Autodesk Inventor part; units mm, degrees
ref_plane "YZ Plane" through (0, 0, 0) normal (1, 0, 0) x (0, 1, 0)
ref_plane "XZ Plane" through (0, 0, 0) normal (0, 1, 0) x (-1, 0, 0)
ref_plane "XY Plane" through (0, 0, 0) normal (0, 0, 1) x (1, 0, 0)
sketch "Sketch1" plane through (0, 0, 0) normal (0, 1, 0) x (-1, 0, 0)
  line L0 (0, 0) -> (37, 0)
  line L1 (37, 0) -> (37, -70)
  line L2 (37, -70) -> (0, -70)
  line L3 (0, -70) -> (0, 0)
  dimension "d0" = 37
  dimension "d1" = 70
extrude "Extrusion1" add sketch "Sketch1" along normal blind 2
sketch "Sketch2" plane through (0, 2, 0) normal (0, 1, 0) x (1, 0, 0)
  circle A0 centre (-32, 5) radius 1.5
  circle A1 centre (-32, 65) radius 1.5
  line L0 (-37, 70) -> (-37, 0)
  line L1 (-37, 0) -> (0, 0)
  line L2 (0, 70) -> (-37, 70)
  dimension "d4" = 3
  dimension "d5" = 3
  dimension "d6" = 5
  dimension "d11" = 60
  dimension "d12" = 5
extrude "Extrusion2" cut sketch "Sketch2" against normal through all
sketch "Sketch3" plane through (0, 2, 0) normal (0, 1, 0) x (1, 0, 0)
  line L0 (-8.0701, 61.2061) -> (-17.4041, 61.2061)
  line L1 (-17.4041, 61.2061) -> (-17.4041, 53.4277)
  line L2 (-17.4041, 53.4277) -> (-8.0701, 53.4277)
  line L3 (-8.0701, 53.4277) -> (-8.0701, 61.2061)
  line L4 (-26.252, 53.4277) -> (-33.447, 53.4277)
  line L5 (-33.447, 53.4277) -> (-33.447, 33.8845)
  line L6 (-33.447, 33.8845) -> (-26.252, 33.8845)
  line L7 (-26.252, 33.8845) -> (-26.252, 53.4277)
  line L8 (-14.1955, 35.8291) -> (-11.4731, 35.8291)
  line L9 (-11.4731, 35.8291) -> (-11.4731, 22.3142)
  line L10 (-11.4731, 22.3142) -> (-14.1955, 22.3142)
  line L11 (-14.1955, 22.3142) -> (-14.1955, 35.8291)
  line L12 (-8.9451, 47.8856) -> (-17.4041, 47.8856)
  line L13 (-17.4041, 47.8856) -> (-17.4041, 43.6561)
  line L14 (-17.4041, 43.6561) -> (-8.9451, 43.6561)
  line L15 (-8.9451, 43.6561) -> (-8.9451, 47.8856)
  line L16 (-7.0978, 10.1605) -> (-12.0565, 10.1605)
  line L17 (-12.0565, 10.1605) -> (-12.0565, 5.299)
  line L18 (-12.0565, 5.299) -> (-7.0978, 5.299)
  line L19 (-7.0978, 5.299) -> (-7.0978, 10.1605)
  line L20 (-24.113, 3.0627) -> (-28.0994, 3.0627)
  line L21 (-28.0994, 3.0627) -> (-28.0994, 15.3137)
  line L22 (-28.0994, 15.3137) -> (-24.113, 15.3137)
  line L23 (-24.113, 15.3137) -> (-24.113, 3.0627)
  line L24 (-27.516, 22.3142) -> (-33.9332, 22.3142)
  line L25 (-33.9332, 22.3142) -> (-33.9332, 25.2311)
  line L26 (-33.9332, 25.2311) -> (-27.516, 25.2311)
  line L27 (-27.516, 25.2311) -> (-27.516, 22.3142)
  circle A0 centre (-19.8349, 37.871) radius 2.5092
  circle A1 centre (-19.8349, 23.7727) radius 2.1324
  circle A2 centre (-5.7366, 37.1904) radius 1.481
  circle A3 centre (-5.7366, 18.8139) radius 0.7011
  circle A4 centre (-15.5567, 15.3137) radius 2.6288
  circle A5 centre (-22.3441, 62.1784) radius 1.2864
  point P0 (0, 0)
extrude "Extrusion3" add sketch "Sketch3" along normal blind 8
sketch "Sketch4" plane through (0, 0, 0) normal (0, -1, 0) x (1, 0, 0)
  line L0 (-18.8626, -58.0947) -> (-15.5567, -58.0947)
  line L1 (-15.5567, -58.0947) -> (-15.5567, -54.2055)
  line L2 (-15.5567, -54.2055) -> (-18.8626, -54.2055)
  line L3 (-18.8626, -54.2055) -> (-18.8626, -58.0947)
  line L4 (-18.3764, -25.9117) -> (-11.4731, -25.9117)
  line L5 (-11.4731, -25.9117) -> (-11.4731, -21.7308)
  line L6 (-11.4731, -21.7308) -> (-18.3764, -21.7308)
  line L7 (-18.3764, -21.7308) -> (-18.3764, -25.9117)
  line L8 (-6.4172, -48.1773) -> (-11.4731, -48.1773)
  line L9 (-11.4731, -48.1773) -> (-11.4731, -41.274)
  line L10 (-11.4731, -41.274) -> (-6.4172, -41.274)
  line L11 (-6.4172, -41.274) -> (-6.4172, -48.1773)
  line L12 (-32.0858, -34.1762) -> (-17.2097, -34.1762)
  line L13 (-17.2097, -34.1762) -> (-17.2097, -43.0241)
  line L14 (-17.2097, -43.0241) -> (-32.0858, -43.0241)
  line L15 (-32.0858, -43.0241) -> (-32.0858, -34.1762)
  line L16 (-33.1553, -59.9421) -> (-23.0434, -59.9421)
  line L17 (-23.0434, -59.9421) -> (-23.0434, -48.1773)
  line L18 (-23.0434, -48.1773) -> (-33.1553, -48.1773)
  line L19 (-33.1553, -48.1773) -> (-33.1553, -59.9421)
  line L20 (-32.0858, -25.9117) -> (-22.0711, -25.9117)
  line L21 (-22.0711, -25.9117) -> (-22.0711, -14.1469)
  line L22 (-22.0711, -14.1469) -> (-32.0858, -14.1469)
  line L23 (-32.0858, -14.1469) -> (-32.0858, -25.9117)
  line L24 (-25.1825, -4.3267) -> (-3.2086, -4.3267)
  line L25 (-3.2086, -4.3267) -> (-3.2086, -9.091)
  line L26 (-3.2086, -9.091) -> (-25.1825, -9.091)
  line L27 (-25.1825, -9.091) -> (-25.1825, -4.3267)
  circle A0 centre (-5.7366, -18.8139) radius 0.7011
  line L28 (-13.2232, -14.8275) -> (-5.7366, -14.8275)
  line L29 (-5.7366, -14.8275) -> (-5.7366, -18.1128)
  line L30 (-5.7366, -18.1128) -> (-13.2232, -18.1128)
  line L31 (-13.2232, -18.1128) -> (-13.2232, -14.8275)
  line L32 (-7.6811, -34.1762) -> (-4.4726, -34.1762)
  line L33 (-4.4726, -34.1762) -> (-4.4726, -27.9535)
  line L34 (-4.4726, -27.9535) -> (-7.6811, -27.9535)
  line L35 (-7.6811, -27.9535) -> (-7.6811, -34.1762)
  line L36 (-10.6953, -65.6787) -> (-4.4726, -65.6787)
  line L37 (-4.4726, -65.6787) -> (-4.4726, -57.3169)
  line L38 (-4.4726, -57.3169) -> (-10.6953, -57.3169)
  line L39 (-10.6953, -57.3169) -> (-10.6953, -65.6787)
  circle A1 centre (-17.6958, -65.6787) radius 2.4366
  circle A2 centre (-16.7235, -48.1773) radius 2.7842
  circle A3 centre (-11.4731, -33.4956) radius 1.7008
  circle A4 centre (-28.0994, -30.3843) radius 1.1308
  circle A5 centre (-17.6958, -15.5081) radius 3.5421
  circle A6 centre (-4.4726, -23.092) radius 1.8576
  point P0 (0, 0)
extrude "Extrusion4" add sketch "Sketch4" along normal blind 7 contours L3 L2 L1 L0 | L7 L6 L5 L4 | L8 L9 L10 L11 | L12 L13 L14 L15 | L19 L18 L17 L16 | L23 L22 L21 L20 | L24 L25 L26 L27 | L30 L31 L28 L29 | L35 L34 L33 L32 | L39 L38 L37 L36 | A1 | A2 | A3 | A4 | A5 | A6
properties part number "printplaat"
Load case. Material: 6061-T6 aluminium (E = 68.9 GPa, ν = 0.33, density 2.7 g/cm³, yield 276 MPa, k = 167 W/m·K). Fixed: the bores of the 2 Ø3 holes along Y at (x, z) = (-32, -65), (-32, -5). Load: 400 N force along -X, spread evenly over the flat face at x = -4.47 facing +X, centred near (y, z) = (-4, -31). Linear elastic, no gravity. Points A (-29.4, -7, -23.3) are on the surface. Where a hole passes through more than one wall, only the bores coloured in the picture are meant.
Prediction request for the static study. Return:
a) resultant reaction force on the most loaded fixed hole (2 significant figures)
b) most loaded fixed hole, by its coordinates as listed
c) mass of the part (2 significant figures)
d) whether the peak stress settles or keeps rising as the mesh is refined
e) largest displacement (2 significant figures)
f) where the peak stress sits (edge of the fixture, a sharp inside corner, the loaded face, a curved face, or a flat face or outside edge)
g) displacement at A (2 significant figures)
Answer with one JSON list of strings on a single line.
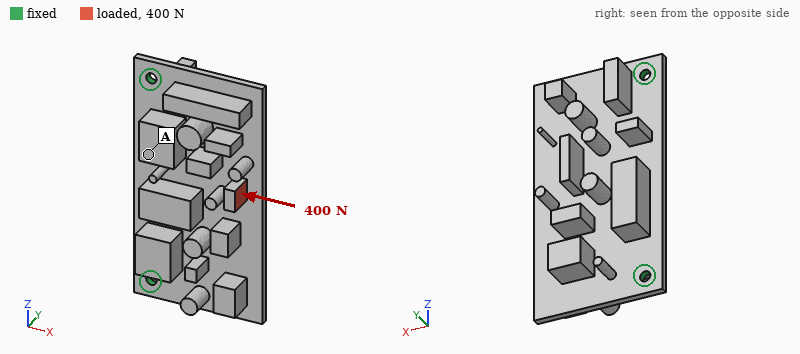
["250 N", "(-32, -5)", "38 g", "keeps rising", "0.27 mm", "edge of the fixture", "0.046 mm"]
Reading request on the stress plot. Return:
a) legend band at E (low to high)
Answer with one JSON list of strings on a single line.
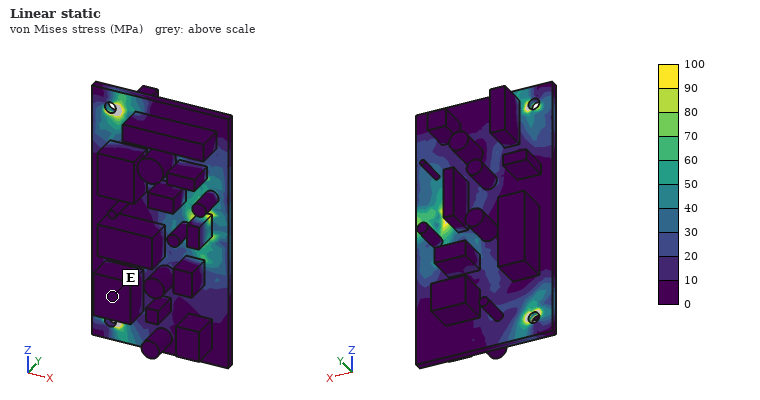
["0 to 10 MPa"]
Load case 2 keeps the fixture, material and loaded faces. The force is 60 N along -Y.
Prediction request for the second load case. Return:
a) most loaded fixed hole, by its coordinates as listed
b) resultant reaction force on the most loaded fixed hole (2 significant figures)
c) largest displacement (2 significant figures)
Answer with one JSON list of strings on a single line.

["(-32, -5)", "38 N", "0.21 mm"]
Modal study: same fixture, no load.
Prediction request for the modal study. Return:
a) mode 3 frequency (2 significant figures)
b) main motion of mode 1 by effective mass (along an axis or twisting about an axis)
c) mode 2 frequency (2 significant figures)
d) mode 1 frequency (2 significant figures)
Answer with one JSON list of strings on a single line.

["2400 Hz", "along Y", "2200 Hz", "920 Hz"]
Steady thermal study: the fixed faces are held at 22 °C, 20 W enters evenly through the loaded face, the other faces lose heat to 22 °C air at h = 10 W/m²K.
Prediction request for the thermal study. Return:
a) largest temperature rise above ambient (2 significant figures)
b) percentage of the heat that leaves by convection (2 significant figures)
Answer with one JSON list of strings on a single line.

["72 K", "10 %"]
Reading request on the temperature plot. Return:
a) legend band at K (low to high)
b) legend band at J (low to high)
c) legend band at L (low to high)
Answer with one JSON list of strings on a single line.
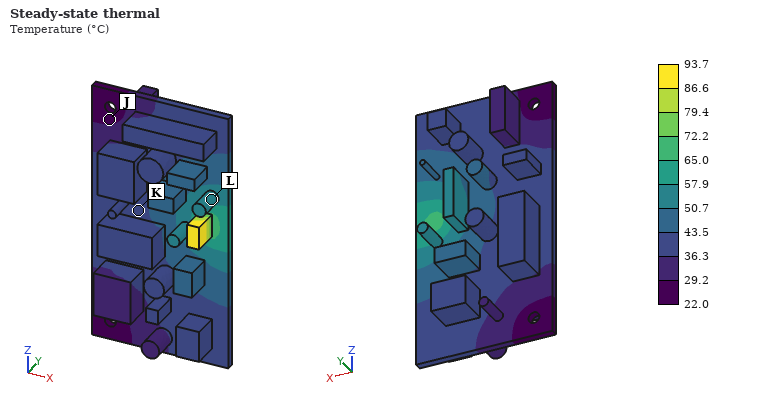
["36.3 to 43.5 °C", "22.0 to 29.2 °C", "50.7 to 57.9 °C"]
